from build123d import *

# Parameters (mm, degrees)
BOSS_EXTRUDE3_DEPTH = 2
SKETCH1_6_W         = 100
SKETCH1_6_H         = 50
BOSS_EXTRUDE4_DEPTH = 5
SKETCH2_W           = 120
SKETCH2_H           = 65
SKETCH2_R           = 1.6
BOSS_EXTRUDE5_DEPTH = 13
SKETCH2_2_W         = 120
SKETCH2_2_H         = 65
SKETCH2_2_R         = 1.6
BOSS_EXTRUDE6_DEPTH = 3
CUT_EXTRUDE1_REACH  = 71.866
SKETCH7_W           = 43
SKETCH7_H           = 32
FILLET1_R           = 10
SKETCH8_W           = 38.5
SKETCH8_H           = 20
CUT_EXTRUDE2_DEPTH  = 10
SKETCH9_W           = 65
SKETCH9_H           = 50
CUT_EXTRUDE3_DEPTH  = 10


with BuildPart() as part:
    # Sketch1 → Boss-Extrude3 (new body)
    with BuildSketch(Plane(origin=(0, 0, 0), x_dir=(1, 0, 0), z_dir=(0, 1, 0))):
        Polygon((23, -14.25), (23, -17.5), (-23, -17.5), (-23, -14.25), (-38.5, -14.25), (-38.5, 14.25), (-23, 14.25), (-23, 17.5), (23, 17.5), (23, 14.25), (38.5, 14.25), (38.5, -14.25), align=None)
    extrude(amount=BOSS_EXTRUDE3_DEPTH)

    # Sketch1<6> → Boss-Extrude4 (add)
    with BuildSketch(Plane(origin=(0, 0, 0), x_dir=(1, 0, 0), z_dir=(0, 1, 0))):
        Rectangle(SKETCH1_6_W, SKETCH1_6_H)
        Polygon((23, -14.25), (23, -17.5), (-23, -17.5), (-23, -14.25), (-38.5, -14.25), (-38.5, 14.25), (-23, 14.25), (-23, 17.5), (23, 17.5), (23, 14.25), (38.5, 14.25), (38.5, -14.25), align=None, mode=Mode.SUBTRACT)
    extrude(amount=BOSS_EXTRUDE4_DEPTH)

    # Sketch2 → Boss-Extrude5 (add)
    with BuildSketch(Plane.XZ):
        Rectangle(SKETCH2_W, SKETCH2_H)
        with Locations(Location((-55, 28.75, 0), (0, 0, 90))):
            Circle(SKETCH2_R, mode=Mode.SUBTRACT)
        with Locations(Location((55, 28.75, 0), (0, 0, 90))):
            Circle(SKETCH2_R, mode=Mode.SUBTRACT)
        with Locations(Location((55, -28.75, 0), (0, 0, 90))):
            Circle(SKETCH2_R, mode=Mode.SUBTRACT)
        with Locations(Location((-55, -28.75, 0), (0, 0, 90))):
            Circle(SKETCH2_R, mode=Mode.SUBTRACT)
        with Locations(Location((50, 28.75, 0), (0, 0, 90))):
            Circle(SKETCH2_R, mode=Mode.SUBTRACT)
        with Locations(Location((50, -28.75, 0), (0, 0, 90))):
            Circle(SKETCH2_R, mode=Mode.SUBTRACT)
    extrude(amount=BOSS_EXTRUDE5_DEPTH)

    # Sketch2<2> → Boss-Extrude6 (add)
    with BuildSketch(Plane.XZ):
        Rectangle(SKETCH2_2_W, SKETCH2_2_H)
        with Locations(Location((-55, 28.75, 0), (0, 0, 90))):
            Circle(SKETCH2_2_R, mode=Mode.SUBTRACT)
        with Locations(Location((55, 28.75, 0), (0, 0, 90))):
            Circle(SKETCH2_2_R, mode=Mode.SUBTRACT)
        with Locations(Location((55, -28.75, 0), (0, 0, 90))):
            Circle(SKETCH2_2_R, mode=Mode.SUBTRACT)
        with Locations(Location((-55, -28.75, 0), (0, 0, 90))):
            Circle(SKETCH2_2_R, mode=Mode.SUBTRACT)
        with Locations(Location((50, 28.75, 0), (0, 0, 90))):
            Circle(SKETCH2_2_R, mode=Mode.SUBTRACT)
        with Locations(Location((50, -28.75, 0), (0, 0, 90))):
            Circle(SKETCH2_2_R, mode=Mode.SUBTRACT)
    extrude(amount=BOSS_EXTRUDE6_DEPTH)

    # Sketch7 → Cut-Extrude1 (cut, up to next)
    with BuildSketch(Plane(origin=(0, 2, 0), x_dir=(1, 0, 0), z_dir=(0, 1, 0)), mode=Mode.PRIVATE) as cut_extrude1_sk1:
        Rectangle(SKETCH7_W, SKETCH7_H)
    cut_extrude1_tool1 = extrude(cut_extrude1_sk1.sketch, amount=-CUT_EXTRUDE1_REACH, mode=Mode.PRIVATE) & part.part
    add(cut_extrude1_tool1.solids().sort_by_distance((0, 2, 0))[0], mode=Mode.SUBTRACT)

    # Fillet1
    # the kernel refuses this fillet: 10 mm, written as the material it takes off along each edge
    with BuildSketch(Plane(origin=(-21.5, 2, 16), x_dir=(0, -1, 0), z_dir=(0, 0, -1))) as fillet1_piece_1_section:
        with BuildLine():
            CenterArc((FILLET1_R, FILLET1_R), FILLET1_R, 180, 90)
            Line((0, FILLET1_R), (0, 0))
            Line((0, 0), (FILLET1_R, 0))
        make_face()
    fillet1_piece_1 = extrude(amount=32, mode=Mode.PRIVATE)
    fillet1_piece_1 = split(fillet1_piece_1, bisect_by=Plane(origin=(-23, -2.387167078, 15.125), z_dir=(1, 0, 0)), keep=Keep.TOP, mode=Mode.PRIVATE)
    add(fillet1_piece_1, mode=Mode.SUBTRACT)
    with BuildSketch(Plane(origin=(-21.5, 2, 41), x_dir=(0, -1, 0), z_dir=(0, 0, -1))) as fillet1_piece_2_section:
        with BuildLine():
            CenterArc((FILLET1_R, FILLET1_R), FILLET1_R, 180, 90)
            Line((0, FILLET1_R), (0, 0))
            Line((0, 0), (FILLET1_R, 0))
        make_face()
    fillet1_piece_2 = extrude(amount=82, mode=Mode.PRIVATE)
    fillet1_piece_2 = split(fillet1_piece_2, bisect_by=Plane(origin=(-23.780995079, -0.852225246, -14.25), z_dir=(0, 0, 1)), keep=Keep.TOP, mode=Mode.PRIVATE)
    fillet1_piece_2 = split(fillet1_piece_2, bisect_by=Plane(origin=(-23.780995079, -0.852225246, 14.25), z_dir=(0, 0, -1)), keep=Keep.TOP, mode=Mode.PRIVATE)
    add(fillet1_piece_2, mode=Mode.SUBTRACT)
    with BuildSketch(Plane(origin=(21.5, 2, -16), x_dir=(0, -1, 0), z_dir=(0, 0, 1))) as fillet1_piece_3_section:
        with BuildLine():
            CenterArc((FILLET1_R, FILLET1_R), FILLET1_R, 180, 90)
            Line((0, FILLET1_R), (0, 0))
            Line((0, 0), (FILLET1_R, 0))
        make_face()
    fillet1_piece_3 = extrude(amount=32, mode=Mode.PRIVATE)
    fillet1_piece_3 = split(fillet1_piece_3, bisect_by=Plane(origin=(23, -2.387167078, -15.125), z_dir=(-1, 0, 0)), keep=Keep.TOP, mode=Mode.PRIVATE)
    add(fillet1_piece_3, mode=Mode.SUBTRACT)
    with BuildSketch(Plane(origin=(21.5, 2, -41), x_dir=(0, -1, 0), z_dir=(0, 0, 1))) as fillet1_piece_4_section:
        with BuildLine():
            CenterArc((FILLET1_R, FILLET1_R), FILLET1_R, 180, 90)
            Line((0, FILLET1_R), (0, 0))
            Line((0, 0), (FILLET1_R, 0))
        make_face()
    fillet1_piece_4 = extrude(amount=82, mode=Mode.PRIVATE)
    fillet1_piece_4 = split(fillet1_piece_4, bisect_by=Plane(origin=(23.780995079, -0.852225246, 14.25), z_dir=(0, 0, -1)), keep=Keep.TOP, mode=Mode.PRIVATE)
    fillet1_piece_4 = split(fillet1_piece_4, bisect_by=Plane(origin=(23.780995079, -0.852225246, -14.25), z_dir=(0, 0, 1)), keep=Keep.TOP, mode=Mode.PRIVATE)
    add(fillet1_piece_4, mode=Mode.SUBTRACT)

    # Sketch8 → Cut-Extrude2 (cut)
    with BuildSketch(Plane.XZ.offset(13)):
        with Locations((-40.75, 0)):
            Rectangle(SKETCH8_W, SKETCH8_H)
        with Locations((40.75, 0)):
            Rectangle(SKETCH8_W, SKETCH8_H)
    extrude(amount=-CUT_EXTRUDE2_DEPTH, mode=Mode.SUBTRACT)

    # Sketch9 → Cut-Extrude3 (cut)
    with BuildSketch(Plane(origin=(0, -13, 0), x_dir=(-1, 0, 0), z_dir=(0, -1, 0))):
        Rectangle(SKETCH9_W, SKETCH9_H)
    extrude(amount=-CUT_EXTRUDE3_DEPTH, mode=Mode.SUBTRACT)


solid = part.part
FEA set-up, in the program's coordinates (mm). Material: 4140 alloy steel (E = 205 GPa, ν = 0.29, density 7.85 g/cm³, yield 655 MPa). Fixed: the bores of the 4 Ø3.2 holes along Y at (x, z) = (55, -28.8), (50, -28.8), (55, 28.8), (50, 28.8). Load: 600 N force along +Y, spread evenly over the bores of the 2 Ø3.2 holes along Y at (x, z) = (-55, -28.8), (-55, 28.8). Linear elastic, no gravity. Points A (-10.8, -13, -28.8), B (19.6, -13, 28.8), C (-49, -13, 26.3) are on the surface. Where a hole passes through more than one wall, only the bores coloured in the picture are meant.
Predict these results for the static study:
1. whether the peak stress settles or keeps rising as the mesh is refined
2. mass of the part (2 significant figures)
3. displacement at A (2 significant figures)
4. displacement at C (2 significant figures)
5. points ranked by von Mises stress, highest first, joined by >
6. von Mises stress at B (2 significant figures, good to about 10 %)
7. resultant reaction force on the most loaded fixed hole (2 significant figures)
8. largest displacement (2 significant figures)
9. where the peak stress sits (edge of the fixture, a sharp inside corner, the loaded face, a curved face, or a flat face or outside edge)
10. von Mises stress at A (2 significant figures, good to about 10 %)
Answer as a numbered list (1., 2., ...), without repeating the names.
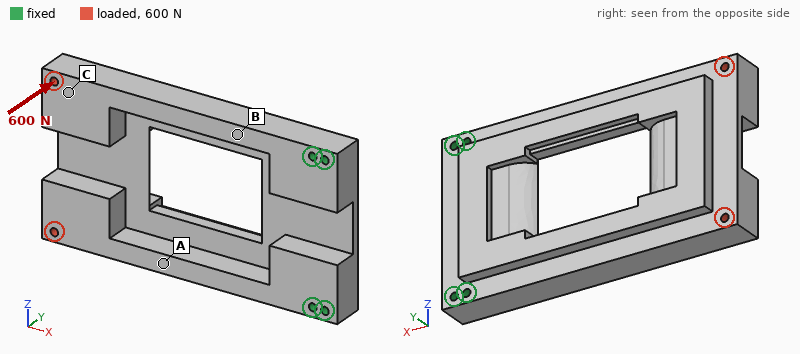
1. keeps rising
2. 520 g
3. 0.068 mm
4. 0.15 mm
5. B > A > C
6. 56 MPa
7. 1.2 kN
8. 0.17 mm
9. edge of the fixture
10. 33 MPa
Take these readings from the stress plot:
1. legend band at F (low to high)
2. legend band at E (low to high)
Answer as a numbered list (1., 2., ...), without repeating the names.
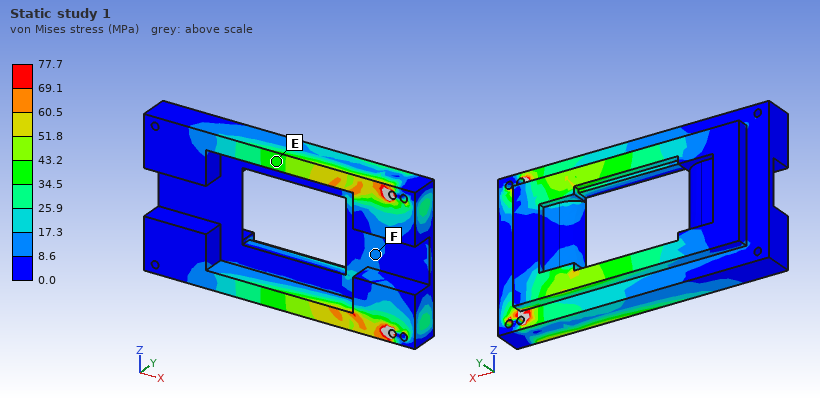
1. 8.6 to 17.3 MPa
2. 34.5 to 43.2 MPa
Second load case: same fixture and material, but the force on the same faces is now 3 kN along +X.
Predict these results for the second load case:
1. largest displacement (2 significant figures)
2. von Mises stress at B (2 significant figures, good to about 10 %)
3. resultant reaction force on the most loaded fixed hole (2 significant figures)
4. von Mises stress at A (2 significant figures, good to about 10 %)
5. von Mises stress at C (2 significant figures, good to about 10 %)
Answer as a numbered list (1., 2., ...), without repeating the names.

1. 28 µm
2. 20 MPa
3. 1.2 kN
4. 20 MPa
5. 9.3 MPa
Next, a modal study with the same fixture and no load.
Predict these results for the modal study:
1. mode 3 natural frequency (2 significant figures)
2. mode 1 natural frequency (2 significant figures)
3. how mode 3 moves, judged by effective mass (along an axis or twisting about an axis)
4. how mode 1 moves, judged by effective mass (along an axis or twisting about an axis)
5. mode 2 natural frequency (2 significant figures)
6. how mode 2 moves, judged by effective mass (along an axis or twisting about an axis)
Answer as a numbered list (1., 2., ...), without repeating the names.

1. 2200 Hz
2. 770 Hz
3. along Z
4. along Y
5. 1300 Hz
6. along Z
